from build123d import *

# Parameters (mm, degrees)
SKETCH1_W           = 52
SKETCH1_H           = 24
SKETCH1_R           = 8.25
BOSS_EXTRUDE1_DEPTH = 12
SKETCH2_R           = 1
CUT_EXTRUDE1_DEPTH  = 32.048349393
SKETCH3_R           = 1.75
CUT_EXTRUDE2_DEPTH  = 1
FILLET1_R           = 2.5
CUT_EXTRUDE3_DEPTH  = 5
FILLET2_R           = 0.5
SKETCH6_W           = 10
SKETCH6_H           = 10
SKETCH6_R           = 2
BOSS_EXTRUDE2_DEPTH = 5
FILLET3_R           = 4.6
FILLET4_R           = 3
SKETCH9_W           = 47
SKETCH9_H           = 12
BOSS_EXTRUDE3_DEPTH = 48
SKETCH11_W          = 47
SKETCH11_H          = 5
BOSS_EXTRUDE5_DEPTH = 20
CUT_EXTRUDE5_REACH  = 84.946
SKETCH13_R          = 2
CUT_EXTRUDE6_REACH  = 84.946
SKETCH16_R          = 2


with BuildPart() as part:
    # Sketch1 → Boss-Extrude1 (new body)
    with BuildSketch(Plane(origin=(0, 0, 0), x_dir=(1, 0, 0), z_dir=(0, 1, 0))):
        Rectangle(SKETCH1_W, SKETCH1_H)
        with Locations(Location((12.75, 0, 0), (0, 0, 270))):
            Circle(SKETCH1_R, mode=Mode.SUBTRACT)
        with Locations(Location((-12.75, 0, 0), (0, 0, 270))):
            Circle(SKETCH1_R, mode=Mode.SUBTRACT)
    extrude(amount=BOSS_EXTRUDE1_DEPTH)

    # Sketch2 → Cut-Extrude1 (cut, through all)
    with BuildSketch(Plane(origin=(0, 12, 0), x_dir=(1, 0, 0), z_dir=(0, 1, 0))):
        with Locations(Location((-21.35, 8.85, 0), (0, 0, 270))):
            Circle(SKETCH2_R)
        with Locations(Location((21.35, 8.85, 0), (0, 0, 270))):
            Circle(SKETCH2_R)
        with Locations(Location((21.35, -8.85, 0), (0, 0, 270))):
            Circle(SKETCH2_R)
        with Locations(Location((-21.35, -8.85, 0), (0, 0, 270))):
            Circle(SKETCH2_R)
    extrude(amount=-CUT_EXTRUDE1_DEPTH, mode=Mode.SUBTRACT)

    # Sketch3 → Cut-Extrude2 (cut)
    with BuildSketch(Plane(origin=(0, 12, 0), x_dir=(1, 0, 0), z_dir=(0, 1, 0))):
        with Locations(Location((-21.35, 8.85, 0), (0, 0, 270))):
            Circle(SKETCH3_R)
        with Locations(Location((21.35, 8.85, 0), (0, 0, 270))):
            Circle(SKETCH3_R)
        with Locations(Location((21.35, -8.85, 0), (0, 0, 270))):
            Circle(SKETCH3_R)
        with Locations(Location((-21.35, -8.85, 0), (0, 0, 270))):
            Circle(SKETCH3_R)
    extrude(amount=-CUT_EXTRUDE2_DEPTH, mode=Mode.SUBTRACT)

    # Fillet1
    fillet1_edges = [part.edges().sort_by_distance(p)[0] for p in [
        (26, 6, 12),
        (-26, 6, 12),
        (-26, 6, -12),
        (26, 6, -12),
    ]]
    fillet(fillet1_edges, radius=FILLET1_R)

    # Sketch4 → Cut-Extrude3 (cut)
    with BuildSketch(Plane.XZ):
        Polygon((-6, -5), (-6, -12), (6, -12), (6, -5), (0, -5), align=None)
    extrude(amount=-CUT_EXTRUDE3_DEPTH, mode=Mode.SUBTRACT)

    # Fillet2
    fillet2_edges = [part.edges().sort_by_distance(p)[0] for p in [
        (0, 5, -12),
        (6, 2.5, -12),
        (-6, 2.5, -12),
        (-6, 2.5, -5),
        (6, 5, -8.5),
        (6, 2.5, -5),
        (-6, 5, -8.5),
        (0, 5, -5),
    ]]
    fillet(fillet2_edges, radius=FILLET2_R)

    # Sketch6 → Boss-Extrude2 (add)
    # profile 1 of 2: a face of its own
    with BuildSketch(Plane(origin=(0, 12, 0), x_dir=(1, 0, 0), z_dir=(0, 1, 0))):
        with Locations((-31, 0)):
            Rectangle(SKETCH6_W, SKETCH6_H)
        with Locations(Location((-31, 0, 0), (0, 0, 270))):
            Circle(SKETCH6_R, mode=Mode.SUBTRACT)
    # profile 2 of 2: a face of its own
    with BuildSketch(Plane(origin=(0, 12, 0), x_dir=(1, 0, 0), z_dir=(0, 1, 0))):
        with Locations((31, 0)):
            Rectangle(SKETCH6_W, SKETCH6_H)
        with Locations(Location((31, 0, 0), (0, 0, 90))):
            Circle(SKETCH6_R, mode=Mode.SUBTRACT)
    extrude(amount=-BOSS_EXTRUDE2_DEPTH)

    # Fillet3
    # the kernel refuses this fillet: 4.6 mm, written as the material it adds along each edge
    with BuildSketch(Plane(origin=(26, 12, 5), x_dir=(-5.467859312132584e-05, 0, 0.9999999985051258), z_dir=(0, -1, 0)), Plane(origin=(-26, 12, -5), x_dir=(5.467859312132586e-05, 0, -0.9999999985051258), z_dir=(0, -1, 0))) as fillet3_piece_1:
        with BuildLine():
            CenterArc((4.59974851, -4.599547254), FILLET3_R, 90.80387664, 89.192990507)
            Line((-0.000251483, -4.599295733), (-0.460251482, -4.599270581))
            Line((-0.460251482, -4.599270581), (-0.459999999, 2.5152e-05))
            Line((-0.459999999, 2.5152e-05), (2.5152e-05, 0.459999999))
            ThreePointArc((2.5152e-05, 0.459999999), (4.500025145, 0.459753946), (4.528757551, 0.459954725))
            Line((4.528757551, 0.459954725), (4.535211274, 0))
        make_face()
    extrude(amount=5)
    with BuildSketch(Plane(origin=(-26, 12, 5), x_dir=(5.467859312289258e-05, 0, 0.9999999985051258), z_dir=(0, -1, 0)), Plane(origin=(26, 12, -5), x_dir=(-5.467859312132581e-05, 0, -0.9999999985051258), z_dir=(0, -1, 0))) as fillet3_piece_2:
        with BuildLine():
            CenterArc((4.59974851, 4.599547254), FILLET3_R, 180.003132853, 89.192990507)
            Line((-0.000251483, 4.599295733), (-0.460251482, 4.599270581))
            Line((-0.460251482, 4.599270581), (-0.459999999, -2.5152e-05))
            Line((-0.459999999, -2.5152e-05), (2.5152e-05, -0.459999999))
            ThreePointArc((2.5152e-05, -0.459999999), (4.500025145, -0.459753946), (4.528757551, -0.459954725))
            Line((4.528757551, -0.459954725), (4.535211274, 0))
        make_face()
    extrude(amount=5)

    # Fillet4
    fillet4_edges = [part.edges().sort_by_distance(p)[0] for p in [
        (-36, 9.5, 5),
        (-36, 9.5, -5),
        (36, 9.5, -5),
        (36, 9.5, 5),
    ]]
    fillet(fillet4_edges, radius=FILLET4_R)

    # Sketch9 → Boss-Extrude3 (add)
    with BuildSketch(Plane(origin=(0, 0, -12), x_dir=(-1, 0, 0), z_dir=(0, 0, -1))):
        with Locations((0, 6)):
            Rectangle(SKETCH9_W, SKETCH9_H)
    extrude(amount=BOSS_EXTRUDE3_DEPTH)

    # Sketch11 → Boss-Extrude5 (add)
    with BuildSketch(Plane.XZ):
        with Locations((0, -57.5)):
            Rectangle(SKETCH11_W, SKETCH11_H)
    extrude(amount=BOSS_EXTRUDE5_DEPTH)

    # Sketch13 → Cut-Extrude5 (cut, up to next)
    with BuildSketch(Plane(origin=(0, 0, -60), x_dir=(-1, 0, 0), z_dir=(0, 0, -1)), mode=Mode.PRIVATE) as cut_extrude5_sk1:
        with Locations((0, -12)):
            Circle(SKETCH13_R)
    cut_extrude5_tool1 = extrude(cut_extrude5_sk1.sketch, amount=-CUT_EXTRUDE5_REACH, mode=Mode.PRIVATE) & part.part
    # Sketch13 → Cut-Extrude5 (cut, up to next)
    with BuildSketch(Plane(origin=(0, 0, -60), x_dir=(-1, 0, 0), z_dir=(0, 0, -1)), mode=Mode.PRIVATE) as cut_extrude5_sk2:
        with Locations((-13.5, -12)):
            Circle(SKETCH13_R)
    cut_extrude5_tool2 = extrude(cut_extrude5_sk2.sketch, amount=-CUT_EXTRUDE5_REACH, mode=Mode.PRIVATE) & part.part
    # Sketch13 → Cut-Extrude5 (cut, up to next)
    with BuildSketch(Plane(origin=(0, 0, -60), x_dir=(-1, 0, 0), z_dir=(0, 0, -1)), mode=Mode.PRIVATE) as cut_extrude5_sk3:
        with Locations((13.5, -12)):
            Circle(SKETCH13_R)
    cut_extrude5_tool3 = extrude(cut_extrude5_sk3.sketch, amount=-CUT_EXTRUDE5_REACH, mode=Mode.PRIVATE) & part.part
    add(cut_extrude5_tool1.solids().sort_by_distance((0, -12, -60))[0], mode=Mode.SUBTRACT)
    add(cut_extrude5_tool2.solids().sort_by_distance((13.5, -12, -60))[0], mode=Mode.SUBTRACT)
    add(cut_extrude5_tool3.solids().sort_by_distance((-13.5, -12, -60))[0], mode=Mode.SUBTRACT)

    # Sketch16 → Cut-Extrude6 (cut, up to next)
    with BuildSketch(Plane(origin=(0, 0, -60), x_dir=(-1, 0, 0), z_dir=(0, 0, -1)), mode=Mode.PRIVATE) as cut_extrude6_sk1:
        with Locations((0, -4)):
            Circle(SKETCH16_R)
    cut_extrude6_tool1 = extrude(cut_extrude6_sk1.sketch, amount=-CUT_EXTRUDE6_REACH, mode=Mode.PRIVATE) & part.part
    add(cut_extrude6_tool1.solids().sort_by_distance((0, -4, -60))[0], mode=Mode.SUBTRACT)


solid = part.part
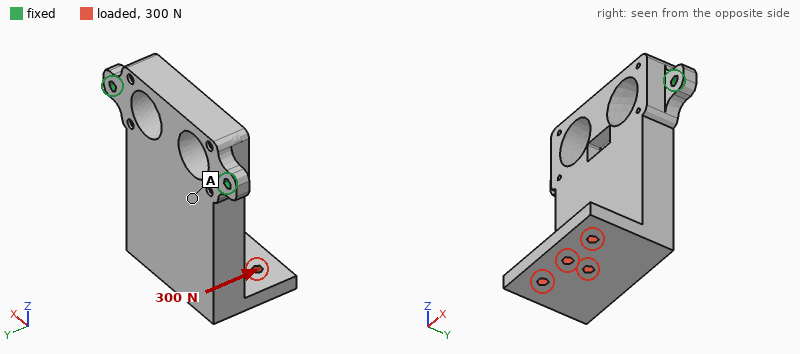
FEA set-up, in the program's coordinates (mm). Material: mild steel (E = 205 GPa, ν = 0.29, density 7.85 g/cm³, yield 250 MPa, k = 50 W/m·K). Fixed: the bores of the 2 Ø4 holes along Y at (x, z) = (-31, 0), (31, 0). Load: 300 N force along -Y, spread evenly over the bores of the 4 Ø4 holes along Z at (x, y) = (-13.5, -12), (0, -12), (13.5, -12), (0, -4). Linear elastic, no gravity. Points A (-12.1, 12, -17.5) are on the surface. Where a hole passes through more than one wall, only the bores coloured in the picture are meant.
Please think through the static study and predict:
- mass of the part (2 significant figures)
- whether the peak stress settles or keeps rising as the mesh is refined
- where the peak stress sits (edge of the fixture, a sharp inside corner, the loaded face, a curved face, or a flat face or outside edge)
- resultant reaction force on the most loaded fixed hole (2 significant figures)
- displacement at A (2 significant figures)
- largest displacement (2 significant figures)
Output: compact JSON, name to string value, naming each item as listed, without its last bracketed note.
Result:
{"mass of the part": "330 g", "whether the peak stress settles or keeps rising as the mesh is refined": "keeps rising", "where the peak stress sits": "edge of the fixture", "resultant reaction force on the most loaded fixed hole": "200 N", "displacement at A": "0.031 mm", "largest displacement": "0.13 mm"}
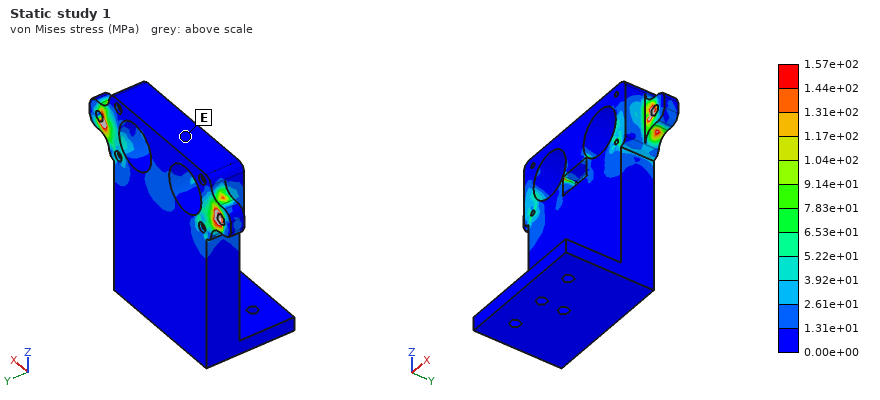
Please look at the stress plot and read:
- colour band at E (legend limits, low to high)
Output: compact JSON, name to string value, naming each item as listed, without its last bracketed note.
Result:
{"colour band at E": "0.00e+00 to 1.31e+01 MPa"}
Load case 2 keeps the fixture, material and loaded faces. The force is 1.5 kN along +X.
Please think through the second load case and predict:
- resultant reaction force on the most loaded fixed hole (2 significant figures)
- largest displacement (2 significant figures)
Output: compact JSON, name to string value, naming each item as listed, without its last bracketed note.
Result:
{"resultant reaction force on the most loaded fixed hole": "1.8 kN", "largest displacement": "36 µm"}
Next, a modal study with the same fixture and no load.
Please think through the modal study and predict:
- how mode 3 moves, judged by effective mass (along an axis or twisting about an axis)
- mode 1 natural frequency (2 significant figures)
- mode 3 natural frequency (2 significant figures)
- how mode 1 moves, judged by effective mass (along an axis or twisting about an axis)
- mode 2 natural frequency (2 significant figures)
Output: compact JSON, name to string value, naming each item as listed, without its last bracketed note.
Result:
{"how mode 3 moves, judged by effective mass": "along X", "mode 1 natural frequency": "720 Hz", "mode 3 natural frequency": "4900 Hz", "how mode 1 moves, judged by effective mass": "along Y", "mode 2 natural frequency": "4300 Hz"}
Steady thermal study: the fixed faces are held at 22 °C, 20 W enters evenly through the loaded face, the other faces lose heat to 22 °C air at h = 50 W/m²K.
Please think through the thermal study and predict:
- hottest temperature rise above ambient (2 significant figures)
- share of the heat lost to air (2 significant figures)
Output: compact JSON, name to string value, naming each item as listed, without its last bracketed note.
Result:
{"hottest temperature rise above ambient": "54 K", "share of the heat lost to air": "70 %"}
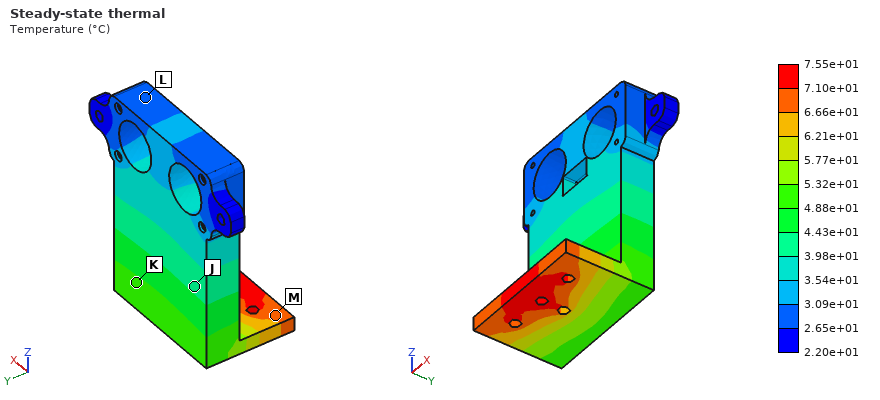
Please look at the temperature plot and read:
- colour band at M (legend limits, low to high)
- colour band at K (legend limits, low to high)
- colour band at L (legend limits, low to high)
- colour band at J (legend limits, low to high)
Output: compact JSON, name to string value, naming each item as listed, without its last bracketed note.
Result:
{"colour band at M": "6.66e+01 to 7.10e+01 °C", "colour band at K": "4.88e+01 to 5.32e+01 °C", "colour band at L": "2.65e+01 to 3.09e+01 °C", "colour band at J": "3.98e+01 to 4.43e+01 °C"}
